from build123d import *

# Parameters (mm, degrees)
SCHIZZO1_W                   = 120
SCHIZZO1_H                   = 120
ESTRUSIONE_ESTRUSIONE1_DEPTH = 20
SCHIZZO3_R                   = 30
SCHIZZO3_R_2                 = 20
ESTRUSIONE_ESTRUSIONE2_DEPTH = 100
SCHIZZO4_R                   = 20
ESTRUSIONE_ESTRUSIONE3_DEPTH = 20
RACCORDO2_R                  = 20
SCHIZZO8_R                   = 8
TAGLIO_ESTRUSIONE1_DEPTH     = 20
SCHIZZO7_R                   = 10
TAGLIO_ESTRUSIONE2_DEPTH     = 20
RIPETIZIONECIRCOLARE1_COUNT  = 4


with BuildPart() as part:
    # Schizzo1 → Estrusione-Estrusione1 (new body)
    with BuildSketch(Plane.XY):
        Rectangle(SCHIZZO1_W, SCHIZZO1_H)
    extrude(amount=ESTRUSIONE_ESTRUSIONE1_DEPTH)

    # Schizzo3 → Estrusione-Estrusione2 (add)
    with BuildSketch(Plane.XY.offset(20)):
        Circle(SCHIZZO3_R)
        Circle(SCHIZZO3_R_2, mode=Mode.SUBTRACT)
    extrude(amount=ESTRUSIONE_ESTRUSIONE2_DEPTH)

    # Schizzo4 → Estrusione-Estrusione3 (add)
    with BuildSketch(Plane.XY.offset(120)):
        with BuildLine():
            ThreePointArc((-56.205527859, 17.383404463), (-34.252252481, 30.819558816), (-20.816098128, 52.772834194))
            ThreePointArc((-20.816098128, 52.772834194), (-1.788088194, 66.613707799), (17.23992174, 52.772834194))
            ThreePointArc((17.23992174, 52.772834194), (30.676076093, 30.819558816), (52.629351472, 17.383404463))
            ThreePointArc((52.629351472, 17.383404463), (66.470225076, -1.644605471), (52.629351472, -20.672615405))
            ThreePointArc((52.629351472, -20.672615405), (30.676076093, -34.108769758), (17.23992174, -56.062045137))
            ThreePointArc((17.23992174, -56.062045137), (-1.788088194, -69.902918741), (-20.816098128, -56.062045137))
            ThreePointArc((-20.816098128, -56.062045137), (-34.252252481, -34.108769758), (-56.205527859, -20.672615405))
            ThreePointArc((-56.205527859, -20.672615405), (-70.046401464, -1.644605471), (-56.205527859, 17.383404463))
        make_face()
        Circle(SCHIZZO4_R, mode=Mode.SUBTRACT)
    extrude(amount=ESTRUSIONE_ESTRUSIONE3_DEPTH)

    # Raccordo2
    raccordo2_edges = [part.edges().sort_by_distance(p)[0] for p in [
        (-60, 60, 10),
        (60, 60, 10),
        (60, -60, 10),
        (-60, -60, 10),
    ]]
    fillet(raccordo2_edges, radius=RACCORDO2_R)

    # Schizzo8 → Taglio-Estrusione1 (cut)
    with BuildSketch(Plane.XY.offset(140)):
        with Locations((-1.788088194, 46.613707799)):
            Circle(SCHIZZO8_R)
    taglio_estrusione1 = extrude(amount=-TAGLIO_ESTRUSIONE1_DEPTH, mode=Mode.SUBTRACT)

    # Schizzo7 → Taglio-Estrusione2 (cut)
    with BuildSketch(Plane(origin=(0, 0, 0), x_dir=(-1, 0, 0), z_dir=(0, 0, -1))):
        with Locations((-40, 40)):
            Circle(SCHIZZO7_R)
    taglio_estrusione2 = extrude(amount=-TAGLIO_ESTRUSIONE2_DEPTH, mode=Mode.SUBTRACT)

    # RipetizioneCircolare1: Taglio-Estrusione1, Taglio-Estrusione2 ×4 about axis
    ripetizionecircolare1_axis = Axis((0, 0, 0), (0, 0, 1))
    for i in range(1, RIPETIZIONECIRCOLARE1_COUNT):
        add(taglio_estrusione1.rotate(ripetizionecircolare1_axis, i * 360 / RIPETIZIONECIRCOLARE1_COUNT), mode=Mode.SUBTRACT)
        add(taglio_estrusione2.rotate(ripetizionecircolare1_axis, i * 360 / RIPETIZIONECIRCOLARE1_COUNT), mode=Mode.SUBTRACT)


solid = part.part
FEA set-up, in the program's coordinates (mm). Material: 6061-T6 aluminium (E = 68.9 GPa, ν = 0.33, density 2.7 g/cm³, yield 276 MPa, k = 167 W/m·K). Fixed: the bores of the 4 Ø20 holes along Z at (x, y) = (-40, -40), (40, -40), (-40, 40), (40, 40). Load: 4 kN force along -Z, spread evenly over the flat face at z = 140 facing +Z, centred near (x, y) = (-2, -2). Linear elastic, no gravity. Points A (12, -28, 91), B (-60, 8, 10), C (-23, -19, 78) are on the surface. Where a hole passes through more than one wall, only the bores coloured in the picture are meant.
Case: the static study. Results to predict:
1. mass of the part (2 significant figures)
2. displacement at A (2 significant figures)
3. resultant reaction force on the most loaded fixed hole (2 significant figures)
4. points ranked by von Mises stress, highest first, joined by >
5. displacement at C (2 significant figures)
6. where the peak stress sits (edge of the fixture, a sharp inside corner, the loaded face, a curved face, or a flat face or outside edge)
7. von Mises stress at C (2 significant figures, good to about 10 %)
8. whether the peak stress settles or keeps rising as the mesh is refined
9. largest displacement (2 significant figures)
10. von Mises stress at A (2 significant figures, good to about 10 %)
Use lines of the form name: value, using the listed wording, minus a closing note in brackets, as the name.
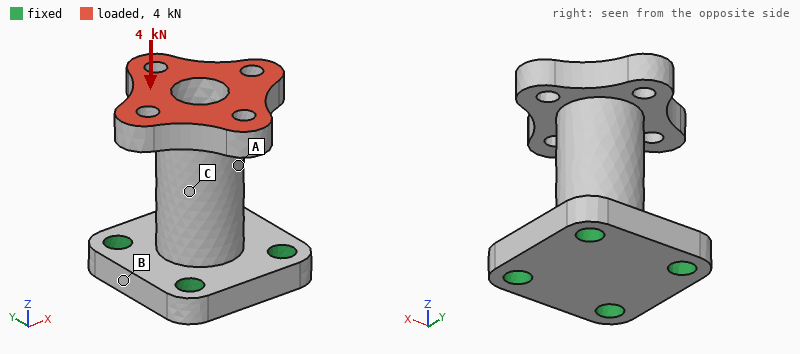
mass of the part: 1.5 kg
displacement at A: 5.3 µm
resultant reaction force on the most loaded fixed hole: 1.2 kN
points ranked by von Mises stress, highest first, joined by >: C > A > B
displacement at C: 5.3 µm
where the peak stress sits: edge of the fixture
von Mises stress at C: 3.2 MPa
whether the peak stress settles or keeps rising as the mesh is refined: keeps rising
largest displacement: 17 µm
von Mises stress at A: 2.4 MPa
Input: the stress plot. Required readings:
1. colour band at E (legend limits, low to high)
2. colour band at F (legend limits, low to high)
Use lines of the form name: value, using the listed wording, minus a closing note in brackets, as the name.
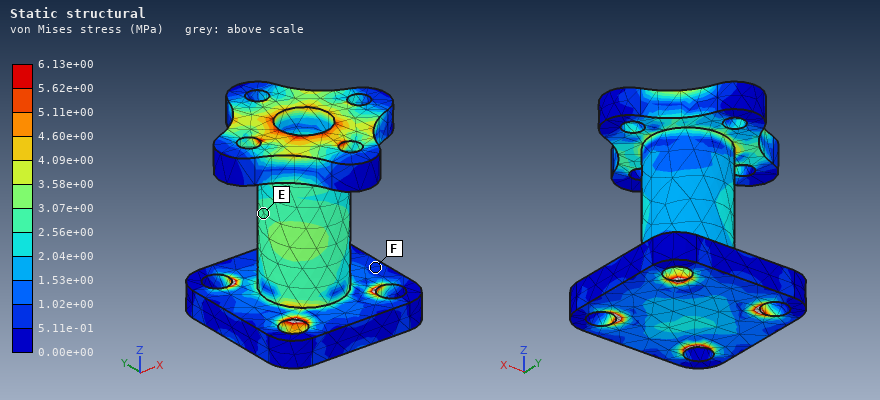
colour band at E: 2.56e+00 to 3.07e+00 MPa
colour band at F: 5.11e-01 to 1.02e+00 MPa
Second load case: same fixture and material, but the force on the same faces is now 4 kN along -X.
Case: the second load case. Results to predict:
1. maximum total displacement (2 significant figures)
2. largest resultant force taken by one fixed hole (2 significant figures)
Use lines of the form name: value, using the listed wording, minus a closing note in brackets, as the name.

maximum total displacement: 0.15 mm
largest resultant force taken by one fixed hole: 4.0 kN
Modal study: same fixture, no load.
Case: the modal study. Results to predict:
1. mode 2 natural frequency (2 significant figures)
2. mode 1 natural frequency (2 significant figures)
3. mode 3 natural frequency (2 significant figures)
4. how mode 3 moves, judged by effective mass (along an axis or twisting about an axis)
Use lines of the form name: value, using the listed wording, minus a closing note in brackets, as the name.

mode 2 natural frequency: 1300 Hz
mode 1 natural frequency: 1300 Hz
mode 3 natural frequency: 2500 Hz
how mode 3 moves, judged by effective mass: twisting about Z
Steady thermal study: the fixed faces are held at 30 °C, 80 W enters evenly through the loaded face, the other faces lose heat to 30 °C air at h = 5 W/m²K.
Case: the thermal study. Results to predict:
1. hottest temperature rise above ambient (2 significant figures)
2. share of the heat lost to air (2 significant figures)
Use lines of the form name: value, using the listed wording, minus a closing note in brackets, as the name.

hottest temperature rise above ambient: 37 K
share of the heat lost to air: 8.4 %
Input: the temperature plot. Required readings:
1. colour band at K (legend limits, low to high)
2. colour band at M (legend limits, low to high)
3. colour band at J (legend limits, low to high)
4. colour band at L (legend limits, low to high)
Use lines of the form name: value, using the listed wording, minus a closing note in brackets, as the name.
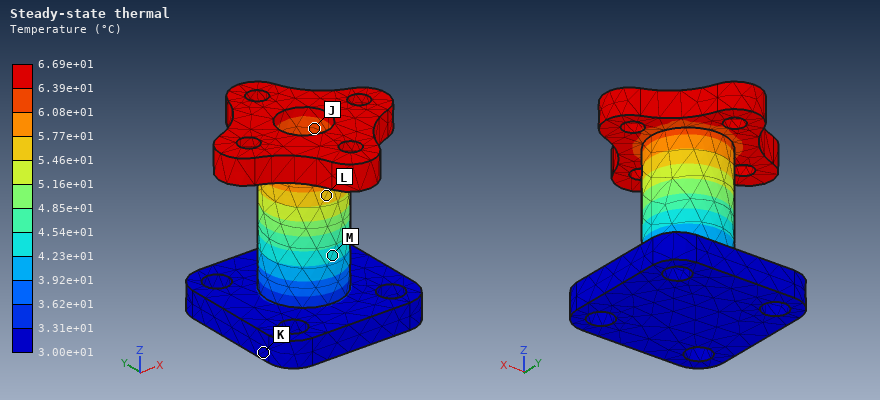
colour band at K: 3.00e+01 to 3.31e+01 °C
colour band at M: 4.23e+01 to 4.54e+01 °C
colour band at J: 6.08e+01 to 6.39e+01 °C
colour band at L: 5.46e+01 to 5.77e+01 °C
